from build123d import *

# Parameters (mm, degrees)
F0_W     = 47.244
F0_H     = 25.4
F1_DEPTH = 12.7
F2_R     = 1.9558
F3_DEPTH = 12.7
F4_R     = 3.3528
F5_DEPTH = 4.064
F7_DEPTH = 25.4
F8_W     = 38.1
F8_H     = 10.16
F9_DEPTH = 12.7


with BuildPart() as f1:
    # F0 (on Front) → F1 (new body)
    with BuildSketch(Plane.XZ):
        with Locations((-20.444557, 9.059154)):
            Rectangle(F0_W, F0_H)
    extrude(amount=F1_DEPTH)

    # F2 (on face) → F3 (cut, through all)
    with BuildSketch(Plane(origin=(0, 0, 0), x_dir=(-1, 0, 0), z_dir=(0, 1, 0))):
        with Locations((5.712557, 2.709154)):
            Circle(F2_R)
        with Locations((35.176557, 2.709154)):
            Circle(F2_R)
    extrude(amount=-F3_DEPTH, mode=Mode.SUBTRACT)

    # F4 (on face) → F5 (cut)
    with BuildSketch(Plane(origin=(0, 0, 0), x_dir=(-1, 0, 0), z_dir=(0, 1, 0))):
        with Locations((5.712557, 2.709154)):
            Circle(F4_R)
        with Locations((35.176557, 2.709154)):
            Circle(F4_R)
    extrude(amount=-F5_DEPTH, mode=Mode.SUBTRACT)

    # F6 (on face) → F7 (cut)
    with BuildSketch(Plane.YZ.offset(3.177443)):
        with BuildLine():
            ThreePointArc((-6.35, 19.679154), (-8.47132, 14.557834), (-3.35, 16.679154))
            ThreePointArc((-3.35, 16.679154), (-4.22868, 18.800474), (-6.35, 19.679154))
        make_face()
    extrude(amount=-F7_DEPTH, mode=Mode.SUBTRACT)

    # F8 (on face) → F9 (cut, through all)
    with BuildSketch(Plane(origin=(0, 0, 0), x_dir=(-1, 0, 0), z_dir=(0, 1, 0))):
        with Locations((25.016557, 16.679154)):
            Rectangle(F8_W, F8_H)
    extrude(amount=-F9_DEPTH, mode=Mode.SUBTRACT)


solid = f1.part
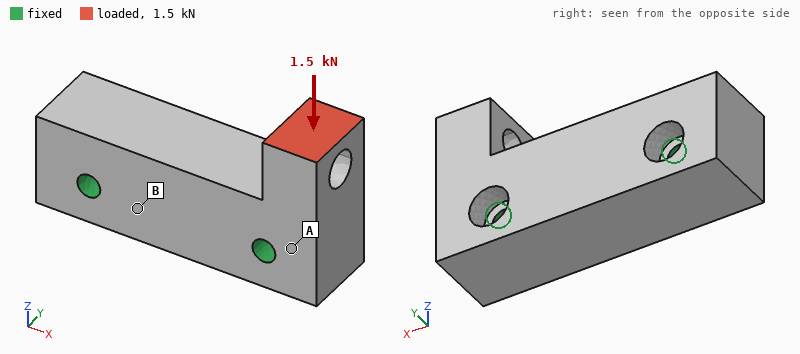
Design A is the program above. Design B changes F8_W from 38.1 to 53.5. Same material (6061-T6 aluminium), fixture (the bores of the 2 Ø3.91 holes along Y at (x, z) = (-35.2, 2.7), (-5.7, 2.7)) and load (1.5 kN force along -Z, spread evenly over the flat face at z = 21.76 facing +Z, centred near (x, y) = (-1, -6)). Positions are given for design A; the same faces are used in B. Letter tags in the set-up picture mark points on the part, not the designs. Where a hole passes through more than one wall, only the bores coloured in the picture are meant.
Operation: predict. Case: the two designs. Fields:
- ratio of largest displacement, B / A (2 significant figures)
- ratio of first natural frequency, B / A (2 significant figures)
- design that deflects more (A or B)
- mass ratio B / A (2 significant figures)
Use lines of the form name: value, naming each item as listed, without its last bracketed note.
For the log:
ratio of largest displacement, B / A: 4.2
ratio of first natural frequency, B / A: 0.51
design that deflects more: B
mass ratio B / A: 0.92
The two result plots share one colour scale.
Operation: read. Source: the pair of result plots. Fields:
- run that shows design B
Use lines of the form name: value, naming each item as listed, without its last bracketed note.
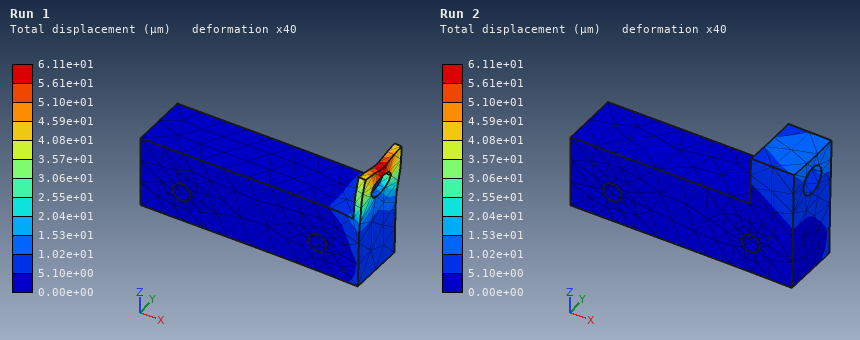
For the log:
run that shows design B: Run 1
